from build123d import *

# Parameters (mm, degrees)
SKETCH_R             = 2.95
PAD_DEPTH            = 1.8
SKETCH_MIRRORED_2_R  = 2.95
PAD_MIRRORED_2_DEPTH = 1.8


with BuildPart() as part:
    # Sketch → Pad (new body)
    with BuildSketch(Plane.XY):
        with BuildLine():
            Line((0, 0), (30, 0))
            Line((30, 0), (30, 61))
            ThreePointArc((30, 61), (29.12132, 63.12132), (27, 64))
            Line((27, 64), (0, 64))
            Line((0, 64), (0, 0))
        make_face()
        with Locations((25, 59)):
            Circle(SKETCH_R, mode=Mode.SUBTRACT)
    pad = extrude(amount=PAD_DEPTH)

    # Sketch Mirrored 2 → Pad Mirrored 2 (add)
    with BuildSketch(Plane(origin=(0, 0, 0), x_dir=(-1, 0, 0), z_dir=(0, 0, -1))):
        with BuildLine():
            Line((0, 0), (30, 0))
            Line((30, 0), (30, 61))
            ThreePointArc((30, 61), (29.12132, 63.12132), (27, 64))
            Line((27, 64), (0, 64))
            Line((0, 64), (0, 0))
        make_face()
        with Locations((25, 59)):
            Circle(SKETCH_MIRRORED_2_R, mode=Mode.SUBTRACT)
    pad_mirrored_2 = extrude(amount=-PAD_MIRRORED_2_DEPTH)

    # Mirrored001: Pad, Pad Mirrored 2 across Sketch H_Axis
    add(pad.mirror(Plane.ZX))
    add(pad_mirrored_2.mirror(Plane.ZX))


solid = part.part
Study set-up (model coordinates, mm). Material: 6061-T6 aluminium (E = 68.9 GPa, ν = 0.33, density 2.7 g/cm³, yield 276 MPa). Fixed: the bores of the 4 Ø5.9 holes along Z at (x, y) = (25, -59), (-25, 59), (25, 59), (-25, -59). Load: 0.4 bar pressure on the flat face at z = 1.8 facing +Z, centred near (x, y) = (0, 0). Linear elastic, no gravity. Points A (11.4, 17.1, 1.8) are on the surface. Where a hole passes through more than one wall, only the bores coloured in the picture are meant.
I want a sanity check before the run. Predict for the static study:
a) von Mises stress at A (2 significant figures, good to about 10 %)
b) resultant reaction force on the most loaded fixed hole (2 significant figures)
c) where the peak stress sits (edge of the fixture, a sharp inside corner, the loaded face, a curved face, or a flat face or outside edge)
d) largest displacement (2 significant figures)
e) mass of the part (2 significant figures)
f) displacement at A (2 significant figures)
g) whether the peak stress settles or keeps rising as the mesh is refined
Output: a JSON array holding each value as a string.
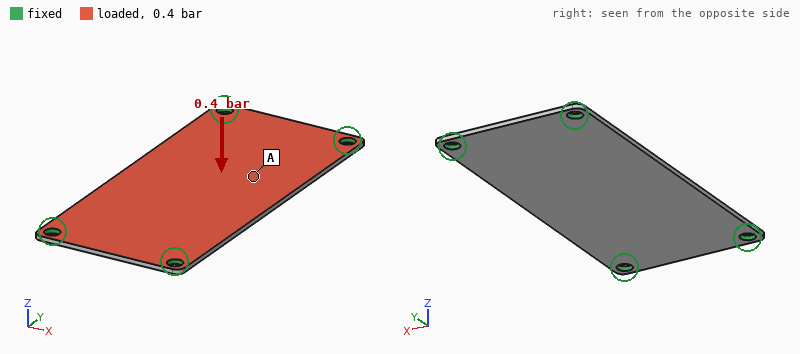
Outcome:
["31 MPa", "76 N", "edge of the fixture", "0.66 mm", "37 g", "0.54 mm", "keeps rising"]
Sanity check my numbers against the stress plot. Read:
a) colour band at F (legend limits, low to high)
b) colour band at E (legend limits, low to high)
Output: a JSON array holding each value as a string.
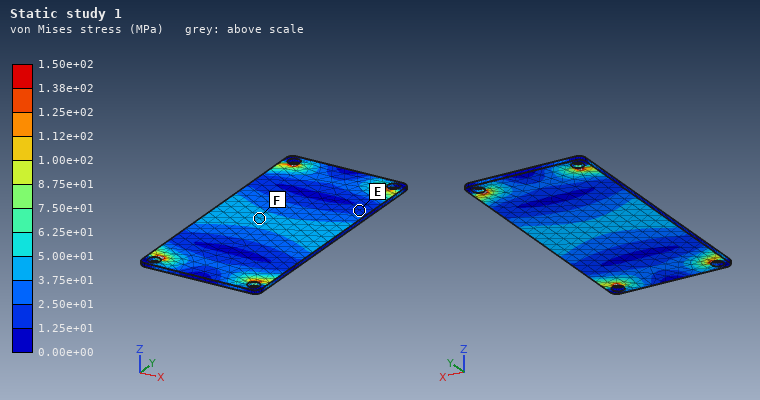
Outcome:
["3.75e+01 to 5.00e+01 MPa", "1.25e+01 to 2.50e+01 MPa"]
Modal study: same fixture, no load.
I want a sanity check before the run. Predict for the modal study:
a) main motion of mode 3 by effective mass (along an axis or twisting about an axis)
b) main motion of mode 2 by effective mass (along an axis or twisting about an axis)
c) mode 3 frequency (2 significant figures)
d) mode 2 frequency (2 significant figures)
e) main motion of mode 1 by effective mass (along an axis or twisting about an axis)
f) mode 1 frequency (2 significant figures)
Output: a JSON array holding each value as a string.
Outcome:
["twisting about X", "twisting about Y", "1800 Hz", "1200 Hz", "along Z", "650 Hz"]
